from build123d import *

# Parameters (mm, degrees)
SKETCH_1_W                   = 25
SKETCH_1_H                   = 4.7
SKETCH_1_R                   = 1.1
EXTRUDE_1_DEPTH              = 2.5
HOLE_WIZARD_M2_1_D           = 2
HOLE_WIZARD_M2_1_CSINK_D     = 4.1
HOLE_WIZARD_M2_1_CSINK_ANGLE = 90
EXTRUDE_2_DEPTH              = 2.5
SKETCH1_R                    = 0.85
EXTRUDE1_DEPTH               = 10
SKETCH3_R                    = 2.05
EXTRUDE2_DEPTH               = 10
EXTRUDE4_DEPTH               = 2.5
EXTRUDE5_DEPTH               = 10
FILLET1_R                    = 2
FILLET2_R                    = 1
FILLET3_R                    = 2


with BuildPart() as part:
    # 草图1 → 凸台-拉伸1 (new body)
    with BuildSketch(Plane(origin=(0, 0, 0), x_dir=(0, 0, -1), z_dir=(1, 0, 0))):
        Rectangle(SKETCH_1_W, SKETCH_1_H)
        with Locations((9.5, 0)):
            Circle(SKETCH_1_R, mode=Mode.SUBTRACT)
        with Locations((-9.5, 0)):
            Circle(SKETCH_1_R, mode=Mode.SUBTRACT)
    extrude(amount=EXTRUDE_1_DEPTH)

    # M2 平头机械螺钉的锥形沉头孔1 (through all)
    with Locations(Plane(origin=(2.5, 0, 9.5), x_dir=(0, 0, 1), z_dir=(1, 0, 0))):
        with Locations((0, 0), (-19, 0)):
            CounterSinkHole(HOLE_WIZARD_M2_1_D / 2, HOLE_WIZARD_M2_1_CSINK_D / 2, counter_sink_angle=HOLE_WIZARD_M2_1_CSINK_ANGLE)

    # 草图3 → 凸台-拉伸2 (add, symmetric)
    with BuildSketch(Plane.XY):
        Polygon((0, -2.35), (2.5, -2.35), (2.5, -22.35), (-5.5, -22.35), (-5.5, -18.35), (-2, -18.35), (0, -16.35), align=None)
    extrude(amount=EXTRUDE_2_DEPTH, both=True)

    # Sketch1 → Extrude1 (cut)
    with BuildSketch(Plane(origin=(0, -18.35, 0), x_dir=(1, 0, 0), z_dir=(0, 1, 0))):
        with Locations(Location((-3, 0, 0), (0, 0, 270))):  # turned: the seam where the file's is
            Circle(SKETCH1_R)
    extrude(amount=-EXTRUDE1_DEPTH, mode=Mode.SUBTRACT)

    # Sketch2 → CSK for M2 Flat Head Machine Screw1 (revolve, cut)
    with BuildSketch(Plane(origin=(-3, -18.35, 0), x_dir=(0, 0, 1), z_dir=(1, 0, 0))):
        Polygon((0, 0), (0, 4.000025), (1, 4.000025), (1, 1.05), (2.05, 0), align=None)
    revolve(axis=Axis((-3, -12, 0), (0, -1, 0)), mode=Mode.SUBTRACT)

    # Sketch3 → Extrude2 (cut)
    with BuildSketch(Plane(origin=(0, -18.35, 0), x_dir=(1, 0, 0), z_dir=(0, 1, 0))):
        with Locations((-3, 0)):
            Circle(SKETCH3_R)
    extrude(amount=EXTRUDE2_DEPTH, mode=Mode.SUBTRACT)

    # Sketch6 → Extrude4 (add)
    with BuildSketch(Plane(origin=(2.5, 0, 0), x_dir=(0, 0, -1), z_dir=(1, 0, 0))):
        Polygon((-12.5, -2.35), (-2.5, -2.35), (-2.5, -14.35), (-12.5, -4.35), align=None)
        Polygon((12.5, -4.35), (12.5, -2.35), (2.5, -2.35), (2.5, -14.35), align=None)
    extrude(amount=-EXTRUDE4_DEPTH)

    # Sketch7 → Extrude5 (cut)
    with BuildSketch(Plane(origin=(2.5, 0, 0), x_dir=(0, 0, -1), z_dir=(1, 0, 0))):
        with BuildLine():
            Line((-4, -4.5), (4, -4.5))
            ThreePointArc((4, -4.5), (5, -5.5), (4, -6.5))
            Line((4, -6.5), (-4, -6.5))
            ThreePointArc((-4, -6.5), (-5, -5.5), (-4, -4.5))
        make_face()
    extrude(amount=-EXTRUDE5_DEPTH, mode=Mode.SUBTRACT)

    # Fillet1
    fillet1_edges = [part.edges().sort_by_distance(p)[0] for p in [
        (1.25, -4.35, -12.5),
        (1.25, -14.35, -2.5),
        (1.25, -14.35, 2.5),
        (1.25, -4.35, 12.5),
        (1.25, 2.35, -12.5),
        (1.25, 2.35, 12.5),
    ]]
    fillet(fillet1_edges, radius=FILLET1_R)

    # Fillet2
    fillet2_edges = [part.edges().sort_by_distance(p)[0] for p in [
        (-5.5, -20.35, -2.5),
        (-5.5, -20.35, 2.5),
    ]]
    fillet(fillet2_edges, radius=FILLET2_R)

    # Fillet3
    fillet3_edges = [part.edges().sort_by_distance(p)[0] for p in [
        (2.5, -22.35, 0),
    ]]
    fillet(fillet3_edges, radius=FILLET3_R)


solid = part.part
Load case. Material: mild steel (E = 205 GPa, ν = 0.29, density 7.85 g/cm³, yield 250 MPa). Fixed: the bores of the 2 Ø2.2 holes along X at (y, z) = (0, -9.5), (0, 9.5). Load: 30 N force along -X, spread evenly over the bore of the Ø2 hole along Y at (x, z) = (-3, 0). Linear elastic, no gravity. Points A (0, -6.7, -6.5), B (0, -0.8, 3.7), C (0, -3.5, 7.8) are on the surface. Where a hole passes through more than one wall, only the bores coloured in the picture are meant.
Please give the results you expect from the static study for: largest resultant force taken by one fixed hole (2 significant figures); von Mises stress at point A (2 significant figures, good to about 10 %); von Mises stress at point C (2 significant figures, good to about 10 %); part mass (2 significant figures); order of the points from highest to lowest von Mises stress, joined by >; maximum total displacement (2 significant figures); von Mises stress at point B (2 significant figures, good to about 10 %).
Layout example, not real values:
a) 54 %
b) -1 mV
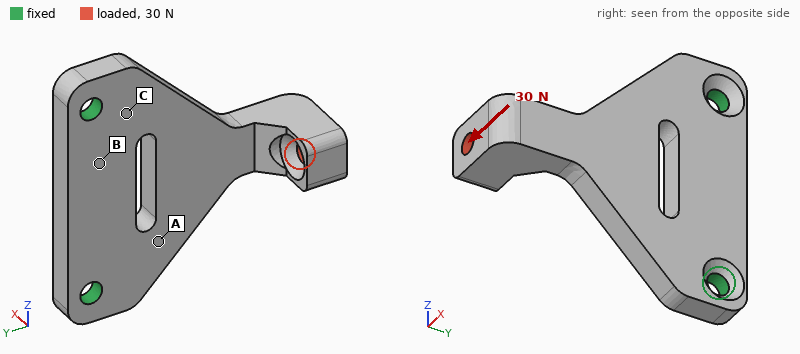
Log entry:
a) 16 N
b) 46 MPa
c) 33 MPa
d) 7.1 g
e) A > C > B
f) 48 µm
g) 9.5 MPa
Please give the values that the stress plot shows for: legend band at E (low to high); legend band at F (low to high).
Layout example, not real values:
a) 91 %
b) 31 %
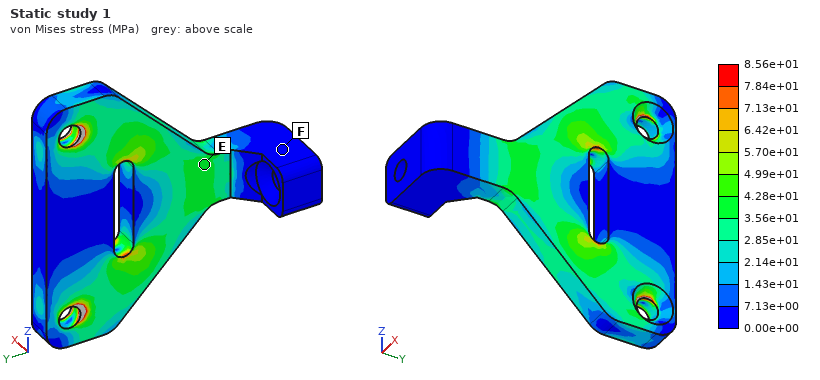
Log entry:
a) 3.56e+01 to 4.28e+01 MPa
b) 0.00e+00 to 7.13e+00 MPa
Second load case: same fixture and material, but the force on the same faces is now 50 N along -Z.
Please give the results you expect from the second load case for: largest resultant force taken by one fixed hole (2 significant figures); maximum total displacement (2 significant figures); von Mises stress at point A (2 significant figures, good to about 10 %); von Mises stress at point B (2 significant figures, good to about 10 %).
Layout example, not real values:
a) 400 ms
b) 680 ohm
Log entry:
a) 59 N
b) 11 µm
c) 9.1 MPa
d) 4.2 MPa
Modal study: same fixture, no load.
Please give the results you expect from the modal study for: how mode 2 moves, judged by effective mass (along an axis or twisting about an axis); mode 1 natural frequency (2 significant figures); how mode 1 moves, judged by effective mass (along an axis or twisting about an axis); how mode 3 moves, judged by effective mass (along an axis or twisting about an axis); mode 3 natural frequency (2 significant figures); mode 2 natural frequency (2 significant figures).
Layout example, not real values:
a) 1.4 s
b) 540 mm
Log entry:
a) along Z
b) 3600 Hz
c) along X
d) along X
e) 15 kHz
f) 14 kHz
